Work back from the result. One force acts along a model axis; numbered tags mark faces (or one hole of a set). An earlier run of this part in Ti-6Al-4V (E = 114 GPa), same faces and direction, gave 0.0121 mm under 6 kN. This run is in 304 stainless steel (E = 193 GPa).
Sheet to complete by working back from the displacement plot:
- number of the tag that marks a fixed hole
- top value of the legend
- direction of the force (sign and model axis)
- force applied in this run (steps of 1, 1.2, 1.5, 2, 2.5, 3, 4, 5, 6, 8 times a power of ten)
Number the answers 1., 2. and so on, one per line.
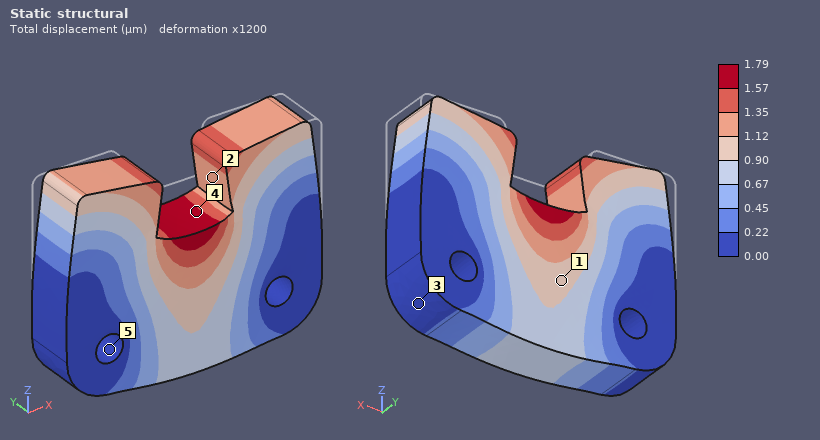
1. 5
2. 1.79 µm
3. -Z
4. 1.5 kN
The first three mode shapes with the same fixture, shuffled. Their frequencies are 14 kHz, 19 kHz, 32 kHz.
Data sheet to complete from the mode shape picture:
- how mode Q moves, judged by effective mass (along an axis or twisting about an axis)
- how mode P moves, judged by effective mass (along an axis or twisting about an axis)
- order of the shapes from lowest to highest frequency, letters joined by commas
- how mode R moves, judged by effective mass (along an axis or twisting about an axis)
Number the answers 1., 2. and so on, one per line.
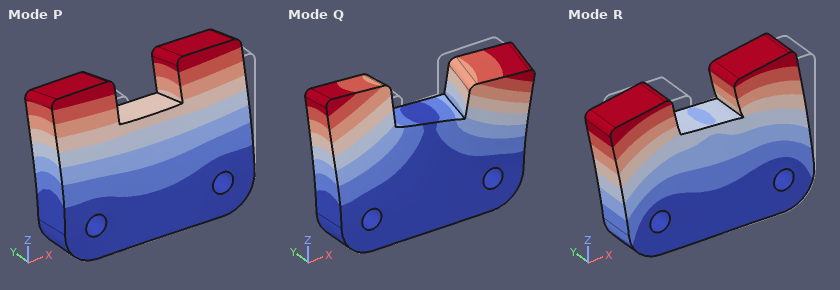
1. twisting about Z
2. along Y
3. P, Q, R
4. along X
